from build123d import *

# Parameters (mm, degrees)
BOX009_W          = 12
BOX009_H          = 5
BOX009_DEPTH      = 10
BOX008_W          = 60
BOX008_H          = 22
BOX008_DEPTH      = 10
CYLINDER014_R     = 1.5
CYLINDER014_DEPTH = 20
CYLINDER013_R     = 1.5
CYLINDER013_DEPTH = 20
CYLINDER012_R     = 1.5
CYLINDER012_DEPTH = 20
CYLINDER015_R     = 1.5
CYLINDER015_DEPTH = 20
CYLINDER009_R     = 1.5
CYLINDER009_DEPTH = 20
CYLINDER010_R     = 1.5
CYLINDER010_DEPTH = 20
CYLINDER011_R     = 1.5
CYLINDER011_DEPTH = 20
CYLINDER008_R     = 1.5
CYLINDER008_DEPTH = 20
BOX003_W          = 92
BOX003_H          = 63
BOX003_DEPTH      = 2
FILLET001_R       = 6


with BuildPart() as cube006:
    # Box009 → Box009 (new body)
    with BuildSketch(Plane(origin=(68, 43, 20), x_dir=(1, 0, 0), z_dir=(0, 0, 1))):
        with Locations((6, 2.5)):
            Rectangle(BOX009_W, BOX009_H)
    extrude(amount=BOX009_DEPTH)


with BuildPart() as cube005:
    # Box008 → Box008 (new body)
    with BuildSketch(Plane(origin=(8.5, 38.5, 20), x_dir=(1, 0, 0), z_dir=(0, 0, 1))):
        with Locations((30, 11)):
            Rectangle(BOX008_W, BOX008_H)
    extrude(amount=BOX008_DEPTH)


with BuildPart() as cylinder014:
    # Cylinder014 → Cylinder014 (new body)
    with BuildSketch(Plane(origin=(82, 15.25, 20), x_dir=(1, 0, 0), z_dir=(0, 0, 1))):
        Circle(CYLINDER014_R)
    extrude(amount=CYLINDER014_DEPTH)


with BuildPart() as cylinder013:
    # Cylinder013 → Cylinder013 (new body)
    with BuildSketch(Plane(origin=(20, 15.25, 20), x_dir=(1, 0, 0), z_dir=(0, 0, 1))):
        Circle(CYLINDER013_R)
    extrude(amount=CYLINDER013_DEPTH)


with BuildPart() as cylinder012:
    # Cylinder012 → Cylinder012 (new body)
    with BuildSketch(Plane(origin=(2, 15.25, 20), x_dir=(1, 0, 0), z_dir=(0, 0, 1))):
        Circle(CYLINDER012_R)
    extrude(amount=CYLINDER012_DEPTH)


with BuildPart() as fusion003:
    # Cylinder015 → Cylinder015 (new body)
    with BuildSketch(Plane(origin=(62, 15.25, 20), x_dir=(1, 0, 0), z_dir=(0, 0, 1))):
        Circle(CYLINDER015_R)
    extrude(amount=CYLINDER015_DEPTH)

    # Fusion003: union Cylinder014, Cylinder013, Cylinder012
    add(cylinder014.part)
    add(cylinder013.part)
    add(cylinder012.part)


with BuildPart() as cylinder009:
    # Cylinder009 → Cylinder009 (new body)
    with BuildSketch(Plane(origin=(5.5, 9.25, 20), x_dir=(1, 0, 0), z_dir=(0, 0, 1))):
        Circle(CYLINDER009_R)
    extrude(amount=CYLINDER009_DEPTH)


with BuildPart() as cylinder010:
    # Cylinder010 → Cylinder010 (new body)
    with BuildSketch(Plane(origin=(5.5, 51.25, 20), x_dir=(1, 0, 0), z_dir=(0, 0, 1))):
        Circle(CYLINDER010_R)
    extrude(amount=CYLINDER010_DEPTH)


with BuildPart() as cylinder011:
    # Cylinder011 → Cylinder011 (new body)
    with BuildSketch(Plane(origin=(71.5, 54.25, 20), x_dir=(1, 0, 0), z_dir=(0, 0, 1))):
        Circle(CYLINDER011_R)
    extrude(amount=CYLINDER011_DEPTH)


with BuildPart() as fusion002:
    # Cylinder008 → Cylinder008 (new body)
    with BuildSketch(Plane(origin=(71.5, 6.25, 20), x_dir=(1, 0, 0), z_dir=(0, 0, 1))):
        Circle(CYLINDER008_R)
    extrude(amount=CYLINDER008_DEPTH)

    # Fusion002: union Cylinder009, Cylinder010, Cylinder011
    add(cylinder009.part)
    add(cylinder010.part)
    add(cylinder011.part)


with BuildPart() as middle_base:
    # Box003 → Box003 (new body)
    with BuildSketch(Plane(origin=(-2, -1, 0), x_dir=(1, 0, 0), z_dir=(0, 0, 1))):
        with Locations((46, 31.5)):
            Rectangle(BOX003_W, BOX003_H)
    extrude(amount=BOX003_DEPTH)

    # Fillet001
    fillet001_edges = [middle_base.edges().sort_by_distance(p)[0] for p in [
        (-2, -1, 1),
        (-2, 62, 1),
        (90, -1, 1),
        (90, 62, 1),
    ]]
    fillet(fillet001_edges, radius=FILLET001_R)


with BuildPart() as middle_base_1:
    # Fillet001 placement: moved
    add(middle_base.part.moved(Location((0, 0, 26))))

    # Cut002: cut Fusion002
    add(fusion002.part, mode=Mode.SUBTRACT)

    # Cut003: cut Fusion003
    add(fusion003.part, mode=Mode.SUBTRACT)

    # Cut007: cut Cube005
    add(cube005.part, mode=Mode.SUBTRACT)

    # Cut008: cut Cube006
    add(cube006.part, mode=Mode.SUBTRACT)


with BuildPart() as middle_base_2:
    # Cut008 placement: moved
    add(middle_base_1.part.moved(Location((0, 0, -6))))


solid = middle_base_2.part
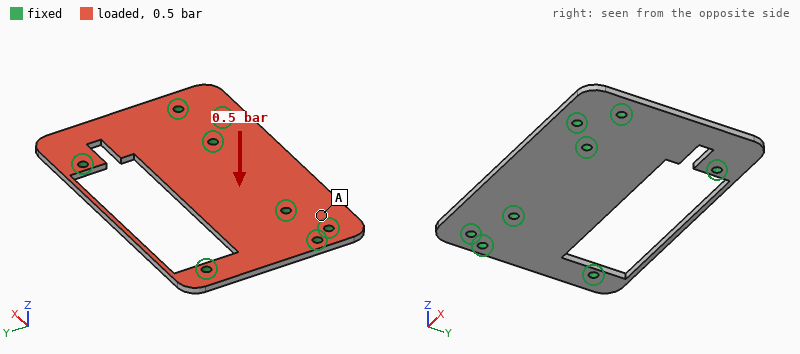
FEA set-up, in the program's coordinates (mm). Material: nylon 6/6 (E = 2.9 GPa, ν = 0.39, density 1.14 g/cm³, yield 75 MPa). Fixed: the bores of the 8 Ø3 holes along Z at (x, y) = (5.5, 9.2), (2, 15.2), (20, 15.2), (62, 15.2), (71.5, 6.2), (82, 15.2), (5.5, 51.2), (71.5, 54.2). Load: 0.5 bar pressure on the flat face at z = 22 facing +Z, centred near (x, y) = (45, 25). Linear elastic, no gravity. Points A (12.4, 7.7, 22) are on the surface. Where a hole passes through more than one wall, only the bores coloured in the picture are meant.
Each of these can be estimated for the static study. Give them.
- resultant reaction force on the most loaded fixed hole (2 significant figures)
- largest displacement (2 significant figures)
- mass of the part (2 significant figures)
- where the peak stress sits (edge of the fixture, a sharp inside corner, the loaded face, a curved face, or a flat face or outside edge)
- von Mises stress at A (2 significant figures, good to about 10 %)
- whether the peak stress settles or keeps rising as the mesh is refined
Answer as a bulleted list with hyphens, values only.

- 61 N
- 1.2 mm
- 9.9 g
- edge of the fixture
- 2.6 MPa
- keeps rising
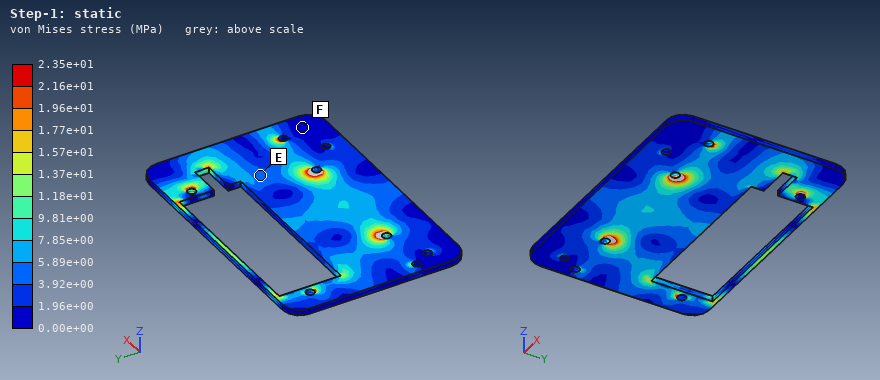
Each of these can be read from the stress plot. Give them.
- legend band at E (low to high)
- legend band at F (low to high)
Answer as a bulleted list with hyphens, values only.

- 3.92e+00 to 5.89e+00 MPa
- 0.00e+00 to 1.96e+00 MPa
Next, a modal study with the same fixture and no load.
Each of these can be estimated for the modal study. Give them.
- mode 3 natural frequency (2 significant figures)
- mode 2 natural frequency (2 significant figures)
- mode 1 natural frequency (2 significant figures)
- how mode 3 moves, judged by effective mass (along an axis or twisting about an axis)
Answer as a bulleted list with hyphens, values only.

- 970 Hz
- 760 Hz
- 650 Hz
- along Z
